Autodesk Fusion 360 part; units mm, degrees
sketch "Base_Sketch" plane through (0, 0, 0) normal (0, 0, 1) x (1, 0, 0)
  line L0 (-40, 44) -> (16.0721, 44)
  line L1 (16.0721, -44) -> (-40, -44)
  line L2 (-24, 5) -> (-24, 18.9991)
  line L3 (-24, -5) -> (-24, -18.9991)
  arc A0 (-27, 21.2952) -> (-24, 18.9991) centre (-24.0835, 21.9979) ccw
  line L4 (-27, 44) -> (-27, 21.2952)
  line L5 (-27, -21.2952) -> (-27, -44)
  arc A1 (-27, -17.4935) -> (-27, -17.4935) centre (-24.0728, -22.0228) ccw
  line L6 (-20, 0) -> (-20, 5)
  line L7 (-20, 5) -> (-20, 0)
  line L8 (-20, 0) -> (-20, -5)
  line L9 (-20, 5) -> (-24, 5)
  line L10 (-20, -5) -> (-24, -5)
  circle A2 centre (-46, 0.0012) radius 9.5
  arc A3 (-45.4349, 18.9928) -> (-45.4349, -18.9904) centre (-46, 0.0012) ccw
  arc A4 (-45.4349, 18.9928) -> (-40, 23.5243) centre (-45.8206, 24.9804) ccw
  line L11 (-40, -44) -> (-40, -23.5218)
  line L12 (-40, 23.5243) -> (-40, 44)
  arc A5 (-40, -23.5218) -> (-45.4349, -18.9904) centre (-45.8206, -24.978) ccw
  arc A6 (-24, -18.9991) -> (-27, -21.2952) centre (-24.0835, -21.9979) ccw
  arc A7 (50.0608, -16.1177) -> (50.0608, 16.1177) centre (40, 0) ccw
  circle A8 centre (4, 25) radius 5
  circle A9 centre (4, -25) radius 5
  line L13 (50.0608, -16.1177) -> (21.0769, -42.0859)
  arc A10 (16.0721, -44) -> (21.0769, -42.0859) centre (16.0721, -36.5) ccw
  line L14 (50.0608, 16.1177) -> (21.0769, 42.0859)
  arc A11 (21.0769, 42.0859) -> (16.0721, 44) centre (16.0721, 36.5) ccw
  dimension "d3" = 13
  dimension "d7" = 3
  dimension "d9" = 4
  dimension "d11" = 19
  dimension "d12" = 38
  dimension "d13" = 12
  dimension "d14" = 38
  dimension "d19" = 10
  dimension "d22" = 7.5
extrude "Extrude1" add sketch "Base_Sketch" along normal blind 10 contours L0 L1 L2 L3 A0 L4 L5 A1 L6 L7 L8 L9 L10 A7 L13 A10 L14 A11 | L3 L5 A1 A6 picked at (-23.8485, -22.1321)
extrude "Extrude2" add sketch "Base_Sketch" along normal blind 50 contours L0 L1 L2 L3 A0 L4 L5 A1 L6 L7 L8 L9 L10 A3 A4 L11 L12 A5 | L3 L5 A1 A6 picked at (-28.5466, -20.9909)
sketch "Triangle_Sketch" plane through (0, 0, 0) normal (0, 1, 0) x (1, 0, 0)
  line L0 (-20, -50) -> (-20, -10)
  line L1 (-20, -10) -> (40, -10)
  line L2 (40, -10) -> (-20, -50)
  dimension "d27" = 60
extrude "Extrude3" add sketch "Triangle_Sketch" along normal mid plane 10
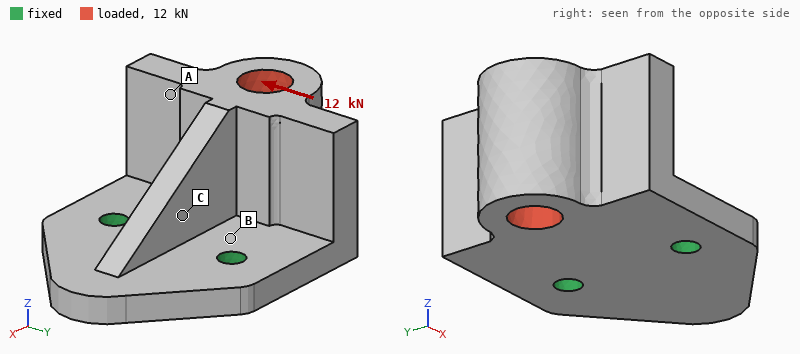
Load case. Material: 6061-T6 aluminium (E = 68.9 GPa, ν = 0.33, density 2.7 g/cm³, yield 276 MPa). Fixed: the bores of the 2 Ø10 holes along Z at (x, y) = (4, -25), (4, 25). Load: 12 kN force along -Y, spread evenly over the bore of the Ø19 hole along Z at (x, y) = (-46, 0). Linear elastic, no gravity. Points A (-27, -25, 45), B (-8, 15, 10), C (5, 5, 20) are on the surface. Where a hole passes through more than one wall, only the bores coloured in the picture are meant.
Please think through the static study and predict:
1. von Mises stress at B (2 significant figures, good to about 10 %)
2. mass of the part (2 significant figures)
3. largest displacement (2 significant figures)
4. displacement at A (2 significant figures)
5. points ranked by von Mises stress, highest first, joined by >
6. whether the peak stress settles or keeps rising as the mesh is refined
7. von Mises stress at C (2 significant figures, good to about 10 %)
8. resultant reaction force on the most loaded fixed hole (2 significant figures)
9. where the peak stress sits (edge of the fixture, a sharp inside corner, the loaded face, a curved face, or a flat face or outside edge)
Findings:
67 MPa
440 g
0.17 mm
0.13 mm
B > C > A
keeps rising
31 MPa
13 kN
edge of the fixture
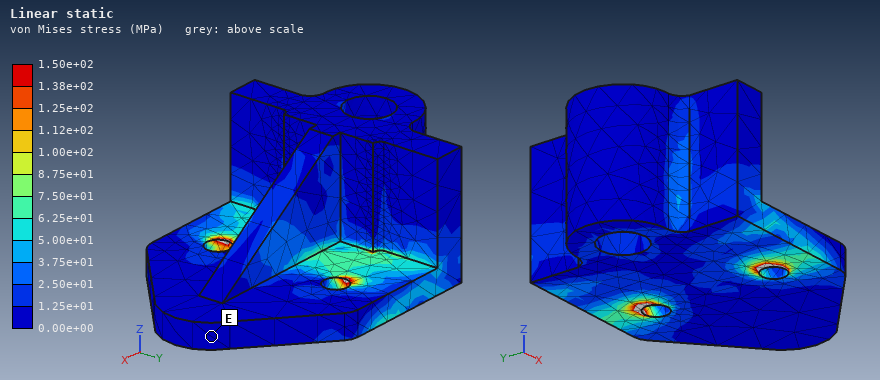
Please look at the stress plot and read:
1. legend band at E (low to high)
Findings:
0.00e+00 to 1.25e+01 MPa
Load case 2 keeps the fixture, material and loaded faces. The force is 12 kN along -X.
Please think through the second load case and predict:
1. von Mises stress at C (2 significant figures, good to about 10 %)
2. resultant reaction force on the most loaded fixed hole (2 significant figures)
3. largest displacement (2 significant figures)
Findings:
36 MPa
6.0 kN
0.34 mm
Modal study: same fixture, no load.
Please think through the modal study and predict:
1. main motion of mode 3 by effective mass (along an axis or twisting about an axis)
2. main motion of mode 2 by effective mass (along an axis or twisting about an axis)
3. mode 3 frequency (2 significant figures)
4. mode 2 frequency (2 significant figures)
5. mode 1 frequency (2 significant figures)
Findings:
along Z
along Y
5300 Hz
2800 Hz
1600 Hz
